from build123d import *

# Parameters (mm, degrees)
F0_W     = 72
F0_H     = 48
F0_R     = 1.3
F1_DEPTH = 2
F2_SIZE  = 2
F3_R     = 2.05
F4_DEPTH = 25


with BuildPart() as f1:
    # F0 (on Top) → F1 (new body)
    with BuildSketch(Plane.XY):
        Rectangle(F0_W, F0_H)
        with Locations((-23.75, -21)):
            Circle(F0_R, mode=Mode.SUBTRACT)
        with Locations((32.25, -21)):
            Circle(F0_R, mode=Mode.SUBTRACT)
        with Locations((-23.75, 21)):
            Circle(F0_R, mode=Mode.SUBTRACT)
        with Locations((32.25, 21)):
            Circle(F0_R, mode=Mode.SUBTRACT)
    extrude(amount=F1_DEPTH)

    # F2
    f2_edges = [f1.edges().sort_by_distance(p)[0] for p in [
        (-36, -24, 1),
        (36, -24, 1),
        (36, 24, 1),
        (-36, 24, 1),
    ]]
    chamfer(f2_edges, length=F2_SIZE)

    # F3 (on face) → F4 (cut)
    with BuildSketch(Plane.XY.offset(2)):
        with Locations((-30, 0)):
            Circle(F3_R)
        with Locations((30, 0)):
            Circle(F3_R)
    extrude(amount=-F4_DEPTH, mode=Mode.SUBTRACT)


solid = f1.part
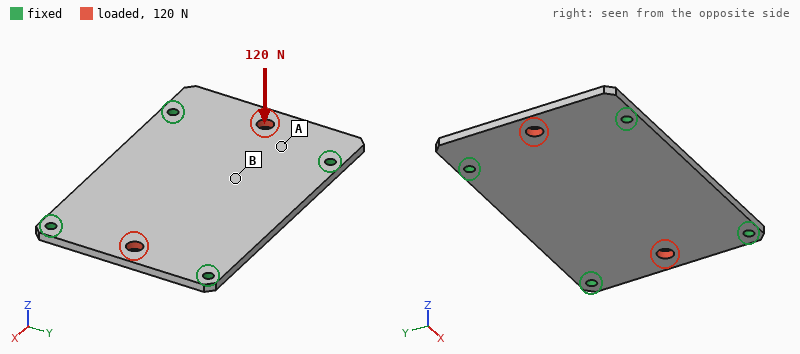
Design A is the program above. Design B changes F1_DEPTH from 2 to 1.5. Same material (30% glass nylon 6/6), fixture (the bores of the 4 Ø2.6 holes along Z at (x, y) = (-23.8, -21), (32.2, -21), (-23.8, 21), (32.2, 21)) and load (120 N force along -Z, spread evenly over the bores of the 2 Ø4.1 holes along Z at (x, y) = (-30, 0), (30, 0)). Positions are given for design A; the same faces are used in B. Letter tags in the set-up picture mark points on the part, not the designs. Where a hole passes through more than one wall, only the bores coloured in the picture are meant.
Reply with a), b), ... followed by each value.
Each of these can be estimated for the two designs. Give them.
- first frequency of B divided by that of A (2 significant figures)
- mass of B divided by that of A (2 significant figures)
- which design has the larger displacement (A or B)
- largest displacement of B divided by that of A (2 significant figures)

a) 0.76
b) 0.75
c) B
d) 2.3
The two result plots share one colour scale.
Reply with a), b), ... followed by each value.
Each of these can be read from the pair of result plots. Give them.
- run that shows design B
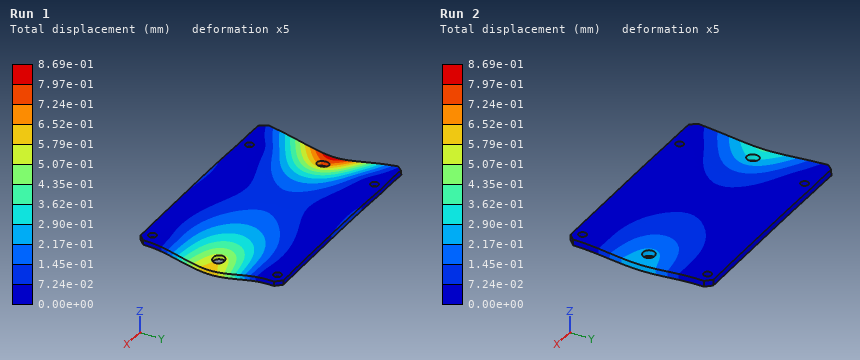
a) Run 1
